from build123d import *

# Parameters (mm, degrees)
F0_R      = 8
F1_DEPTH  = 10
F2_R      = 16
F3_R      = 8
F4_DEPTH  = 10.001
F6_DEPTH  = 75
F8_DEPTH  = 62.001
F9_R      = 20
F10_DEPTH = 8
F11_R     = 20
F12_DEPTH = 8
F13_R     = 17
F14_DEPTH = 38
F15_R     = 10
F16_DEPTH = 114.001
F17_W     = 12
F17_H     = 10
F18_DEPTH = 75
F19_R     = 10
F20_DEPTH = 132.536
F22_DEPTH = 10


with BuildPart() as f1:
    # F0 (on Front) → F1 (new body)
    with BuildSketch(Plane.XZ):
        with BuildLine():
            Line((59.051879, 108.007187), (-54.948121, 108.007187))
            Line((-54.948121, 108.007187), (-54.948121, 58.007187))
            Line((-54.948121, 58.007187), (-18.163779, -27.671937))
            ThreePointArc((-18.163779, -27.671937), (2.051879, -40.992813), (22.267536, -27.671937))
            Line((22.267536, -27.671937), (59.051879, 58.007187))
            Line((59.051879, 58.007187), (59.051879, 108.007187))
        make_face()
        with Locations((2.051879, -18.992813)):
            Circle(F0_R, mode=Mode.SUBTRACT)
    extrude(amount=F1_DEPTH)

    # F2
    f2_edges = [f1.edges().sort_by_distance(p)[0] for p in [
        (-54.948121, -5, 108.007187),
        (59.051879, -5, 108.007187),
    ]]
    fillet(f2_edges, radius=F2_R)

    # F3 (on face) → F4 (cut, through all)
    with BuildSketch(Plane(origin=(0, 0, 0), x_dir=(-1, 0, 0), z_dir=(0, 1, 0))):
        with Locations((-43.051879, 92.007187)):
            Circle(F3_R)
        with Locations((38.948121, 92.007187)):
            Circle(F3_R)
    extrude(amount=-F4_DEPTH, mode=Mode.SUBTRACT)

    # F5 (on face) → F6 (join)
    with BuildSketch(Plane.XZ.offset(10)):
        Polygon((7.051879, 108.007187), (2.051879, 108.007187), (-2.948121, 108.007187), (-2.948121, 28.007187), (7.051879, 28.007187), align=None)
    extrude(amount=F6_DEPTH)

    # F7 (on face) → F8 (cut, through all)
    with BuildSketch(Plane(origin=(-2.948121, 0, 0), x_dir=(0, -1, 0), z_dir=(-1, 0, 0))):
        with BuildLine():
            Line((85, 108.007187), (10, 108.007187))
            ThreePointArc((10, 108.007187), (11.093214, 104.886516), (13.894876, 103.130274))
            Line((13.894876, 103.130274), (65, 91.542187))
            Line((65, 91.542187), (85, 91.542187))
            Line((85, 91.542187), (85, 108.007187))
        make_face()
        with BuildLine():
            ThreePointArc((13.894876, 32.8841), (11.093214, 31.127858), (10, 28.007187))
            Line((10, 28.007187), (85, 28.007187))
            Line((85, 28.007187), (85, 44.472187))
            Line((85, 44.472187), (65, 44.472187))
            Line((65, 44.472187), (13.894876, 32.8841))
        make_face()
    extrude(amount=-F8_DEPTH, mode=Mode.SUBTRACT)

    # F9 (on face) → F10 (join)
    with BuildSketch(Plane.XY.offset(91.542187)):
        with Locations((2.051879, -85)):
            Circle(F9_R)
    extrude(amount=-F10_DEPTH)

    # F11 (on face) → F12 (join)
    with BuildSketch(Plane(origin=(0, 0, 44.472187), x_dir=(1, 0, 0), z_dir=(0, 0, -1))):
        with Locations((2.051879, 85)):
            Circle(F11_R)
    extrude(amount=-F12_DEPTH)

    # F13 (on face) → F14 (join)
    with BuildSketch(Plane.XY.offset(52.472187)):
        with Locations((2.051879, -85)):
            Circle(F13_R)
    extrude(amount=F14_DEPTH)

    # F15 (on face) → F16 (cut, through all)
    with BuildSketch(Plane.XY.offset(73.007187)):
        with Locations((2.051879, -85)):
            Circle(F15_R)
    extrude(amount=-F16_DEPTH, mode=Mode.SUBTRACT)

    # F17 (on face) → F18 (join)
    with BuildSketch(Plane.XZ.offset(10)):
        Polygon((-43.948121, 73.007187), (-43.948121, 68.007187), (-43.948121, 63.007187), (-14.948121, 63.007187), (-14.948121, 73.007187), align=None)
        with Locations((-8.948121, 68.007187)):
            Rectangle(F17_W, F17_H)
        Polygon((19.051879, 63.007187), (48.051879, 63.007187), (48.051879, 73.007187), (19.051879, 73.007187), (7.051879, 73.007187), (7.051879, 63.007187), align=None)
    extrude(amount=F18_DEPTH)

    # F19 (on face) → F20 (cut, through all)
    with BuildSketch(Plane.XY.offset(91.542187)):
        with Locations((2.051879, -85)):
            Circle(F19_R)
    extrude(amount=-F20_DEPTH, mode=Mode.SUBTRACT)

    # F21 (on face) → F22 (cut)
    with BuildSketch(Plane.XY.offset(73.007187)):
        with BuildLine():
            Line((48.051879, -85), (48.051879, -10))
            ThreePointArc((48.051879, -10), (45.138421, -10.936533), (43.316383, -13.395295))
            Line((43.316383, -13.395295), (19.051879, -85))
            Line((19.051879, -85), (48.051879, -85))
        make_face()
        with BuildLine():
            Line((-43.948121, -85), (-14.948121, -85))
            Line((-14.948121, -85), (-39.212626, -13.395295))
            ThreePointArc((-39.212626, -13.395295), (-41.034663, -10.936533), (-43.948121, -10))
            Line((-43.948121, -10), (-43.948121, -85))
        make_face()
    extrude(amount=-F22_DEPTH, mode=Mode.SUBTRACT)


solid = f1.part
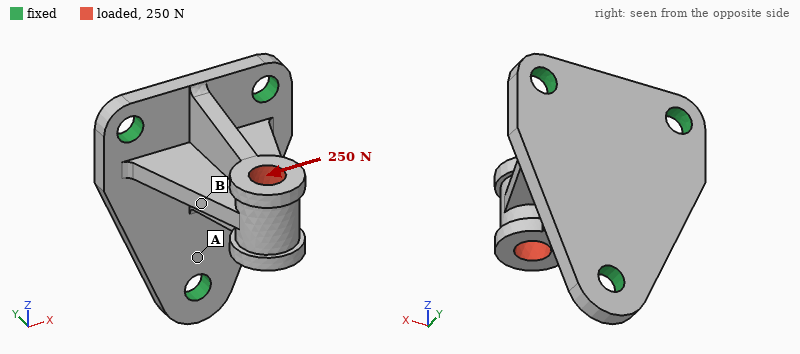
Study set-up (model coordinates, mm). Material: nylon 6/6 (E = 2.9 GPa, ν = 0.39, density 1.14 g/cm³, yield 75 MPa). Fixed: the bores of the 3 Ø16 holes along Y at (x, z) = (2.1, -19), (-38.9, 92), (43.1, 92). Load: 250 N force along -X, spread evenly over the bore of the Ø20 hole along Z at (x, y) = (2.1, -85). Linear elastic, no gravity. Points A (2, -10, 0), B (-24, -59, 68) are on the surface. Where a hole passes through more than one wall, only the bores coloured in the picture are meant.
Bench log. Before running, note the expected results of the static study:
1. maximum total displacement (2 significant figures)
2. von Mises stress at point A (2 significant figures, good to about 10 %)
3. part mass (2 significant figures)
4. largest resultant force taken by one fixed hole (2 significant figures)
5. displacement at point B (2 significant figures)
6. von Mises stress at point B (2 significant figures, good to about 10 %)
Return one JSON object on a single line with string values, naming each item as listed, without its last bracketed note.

{"maximum total displacement": "0.21 mm", "von Mises stress at point A": "0.59 MPa", "part mass": "250 g", "largest resultant force taken by one fixed hole": "280 N", "displacement at point B": "0.10 mm", "von Mises stress at point B": "1.6 MPa"}
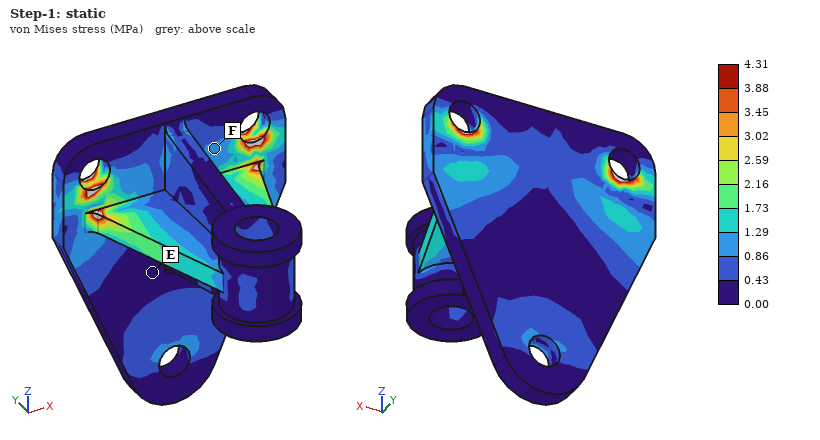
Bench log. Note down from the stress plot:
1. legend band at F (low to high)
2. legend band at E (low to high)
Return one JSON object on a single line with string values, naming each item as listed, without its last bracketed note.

{"legend band at F": "0.86 to 1.29 MPa", "legend band at E": "0.00 to 0.43 MPa"}
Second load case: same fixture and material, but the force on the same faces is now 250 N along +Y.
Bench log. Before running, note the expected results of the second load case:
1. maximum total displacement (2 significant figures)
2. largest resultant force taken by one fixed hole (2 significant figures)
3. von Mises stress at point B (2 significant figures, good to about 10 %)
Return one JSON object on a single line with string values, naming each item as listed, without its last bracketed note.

{"maximum total displacement": "49 µm", "largest resultant force taken by one fixed hole": "110 N", "von Mises stress at point B": "0.33 MPa"}
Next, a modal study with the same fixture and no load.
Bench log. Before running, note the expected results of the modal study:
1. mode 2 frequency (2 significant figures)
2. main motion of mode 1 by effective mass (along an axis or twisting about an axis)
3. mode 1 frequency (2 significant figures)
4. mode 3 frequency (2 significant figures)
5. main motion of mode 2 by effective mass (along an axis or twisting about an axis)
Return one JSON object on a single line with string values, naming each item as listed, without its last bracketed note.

{"mode 2 frequency": "840 Hz", "main motion of mode 1 by effective mass": "along Z", "mode 1 frequency": "560 Hz", "mode 3 frequency": "1200 Hz", "main motion of mode 2 by effective mass": "along X"}
